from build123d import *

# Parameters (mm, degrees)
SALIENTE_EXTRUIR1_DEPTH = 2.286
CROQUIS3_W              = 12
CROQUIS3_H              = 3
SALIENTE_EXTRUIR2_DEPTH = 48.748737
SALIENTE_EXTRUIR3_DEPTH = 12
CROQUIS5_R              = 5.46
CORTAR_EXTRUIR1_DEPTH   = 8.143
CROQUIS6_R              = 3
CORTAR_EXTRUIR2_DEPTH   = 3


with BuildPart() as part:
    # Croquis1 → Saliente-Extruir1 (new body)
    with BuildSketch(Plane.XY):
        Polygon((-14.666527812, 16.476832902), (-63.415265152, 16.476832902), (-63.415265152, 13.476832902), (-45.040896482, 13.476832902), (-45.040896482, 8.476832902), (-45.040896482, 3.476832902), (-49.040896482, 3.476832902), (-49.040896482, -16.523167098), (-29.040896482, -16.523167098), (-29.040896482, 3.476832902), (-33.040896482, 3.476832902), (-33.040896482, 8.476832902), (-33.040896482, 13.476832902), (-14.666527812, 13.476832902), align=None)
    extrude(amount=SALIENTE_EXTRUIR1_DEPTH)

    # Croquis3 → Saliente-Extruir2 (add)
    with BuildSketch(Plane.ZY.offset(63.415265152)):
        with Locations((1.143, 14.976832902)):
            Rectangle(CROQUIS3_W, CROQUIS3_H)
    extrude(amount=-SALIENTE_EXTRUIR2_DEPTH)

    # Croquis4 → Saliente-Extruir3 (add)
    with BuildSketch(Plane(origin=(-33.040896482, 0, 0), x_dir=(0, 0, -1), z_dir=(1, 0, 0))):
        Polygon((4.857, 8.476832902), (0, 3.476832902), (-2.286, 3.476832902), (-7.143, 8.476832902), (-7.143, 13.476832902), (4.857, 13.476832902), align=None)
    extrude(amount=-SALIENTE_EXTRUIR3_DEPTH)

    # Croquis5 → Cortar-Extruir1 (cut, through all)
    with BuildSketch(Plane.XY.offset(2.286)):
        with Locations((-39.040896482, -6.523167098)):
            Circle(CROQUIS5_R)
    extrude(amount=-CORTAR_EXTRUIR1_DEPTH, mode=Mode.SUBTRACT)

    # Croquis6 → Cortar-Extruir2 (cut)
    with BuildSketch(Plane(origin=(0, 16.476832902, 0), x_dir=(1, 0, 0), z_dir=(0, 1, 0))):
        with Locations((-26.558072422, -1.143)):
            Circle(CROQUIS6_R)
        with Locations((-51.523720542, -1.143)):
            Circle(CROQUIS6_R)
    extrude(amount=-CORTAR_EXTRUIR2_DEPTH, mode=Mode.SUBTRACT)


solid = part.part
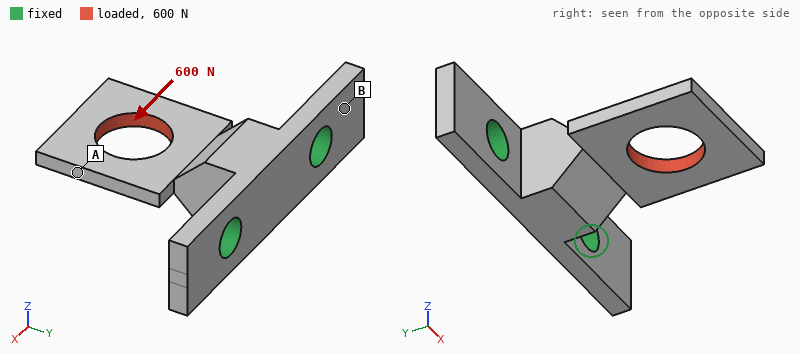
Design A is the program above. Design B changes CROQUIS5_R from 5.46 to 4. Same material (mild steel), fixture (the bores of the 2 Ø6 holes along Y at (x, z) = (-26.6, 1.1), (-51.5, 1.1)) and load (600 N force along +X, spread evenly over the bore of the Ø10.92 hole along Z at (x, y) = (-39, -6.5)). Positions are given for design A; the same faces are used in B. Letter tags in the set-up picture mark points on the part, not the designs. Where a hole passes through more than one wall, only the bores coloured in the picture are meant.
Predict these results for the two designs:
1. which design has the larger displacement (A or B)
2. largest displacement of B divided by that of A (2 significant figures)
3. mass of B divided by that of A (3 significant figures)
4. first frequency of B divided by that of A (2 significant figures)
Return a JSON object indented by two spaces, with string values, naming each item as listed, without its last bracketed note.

{
  "which design has the larger displacement": "A",
  "largest displacement of B divided by that of A": "0.85",
  "mass of B divided by that of A": "1.03",
  "first frequency of B divided by that of A": "1.0"
}
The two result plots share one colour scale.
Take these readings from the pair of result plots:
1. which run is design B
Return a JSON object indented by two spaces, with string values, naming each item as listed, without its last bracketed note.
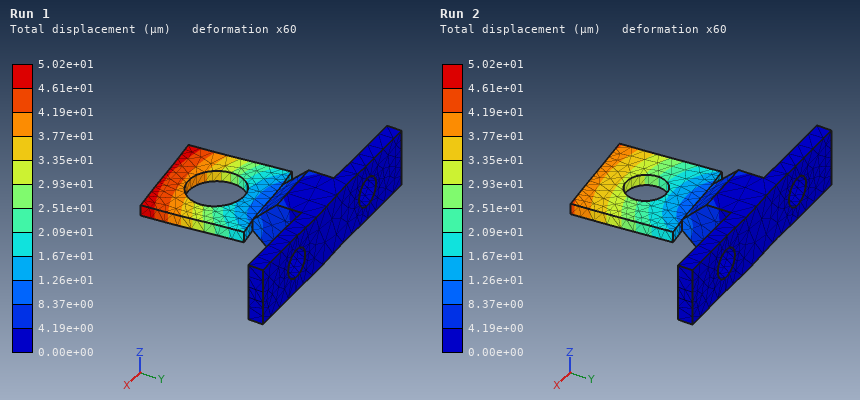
{
  "which run is design B": "Run 2"
}
